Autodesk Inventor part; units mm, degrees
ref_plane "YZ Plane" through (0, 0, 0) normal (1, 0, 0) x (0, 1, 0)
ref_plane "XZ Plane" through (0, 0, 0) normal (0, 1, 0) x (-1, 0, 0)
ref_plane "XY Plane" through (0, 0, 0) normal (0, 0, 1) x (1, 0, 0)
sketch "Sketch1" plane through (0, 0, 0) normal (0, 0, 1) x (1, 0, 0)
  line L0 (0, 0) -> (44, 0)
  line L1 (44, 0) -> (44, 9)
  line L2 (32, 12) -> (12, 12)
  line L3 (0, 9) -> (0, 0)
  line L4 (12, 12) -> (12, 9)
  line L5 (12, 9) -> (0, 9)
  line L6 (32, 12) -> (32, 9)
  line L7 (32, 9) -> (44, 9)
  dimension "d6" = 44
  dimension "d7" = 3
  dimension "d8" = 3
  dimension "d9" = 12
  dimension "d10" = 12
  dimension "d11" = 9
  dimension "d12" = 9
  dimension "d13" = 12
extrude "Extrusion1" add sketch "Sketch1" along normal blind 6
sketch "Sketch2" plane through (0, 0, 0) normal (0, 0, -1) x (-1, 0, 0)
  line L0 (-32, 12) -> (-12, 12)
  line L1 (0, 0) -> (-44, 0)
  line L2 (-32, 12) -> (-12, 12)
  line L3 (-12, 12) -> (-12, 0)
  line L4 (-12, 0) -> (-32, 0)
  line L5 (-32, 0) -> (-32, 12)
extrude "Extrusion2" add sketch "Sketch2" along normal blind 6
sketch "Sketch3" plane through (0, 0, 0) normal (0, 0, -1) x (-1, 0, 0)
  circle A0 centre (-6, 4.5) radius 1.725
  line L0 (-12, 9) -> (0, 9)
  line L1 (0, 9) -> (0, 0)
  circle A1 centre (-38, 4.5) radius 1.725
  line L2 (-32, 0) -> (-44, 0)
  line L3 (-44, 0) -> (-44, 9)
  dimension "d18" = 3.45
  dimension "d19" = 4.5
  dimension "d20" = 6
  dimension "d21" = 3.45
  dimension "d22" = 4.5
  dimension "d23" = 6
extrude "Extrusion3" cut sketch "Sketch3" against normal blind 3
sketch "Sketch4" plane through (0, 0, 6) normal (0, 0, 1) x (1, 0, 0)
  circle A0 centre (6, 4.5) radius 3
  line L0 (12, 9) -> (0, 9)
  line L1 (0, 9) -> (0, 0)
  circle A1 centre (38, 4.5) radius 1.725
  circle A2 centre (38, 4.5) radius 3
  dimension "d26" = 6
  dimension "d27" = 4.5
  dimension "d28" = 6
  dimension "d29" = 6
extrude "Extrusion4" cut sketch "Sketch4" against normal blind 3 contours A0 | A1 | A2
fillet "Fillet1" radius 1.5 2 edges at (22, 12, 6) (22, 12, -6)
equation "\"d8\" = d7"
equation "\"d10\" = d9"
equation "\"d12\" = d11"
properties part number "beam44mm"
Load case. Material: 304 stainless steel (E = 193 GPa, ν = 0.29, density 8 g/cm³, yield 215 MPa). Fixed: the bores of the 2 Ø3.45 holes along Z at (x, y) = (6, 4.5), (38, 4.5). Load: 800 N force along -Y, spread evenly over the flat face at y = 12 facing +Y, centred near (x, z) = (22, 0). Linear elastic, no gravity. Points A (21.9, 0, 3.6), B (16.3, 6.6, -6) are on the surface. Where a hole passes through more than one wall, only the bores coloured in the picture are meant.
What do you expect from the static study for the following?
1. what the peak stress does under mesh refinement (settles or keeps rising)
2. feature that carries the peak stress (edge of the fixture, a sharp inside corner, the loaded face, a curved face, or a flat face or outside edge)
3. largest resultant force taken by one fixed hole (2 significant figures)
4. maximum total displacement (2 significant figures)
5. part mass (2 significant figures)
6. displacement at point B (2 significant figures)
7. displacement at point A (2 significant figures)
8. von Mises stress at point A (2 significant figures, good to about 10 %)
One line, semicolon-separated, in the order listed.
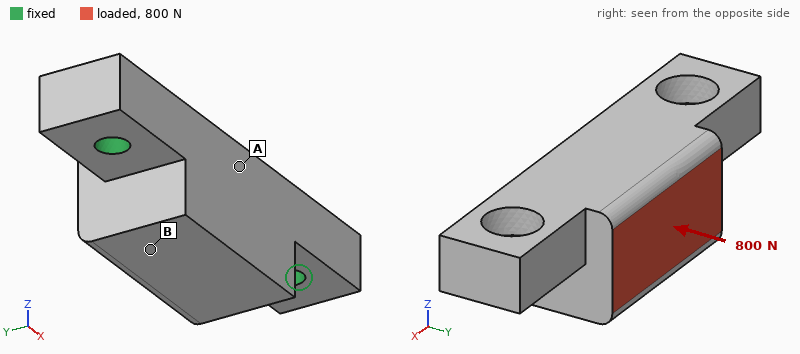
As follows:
keeps rising; edge of the fixture; 410 N; 5.5 µm; 31 g; 4.9 µm; 2.3 µm; 13 MPa
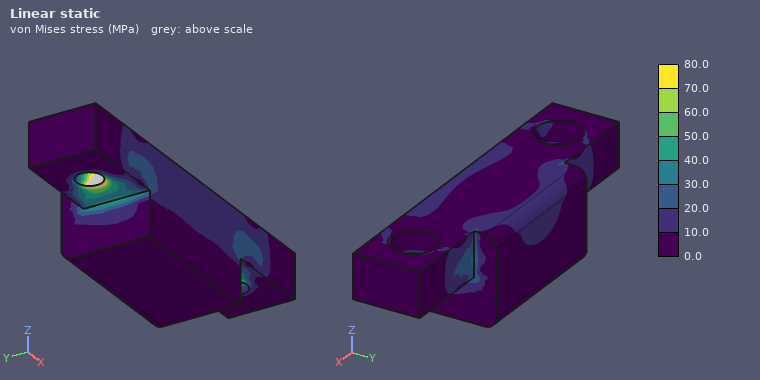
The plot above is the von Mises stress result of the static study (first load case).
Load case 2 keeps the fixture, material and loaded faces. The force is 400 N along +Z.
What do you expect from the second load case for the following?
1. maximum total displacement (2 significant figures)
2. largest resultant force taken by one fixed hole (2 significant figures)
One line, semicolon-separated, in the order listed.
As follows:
7.6 µm; 200 N
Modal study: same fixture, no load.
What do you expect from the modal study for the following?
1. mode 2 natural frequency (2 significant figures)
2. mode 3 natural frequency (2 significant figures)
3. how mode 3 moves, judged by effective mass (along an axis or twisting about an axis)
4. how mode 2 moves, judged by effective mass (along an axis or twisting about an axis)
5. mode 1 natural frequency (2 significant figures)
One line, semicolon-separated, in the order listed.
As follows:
19 kHz; 23 kHz; along Y; along Z; 12 kHz
